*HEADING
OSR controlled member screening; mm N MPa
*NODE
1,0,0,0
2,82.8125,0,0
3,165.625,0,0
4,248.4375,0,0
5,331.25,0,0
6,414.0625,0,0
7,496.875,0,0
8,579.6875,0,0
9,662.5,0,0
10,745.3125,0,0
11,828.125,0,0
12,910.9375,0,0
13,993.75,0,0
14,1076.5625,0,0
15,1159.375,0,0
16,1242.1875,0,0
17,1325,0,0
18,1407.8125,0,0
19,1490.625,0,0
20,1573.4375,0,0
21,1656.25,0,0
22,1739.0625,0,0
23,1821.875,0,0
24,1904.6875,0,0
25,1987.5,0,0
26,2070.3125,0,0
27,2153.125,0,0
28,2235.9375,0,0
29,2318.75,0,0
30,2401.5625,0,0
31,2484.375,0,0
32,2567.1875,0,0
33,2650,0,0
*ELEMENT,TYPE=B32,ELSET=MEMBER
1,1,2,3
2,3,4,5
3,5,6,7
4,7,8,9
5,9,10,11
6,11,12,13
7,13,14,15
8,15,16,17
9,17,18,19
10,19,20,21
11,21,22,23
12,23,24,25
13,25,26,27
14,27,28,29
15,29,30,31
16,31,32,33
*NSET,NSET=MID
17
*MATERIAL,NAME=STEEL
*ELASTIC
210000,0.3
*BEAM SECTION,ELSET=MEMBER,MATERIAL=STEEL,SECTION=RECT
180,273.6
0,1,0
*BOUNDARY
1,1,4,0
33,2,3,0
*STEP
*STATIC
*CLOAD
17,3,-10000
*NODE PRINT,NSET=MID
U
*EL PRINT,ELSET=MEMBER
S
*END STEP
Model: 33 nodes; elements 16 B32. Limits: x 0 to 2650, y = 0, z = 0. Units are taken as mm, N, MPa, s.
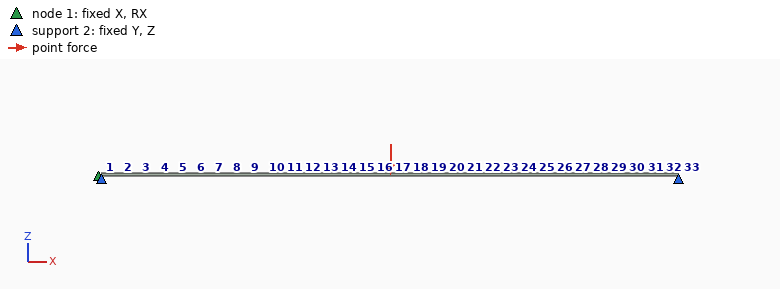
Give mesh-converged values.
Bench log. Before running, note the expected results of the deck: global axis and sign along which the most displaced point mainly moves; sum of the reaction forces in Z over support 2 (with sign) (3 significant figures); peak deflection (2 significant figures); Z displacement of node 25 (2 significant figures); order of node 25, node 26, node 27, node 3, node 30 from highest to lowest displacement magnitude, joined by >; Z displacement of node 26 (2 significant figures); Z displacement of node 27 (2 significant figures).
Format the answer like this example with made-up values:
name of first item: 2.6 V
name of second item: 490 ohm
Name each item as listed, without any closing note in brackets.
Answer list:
global axis and sign along which the most displaced point mainly moves: -Z
sum of the reaction forces in Z over support 2 (with sign): 10000 N
peak deflection: 0.062 mm
Z displacement of node 25: -0.042 mm
order of node 25, node 26, node 27, node 3, node 30 from highest to lowest displacement magnitude, joined by >: node 25 > node 26 > node 27 > node 30 > node 3
Z displacement of node 26: -0.038 mm
Z displacement of node 27: -0.033 mm
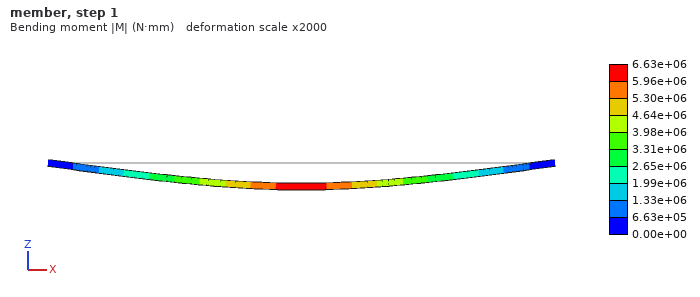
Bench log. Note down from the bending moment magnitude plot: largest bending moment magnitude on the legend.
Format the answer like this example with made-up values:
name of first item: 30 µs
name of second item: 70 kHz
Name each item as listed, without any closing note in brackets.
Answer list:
largest bending moment magnitude on the legend: 6.63e+06 N·mm
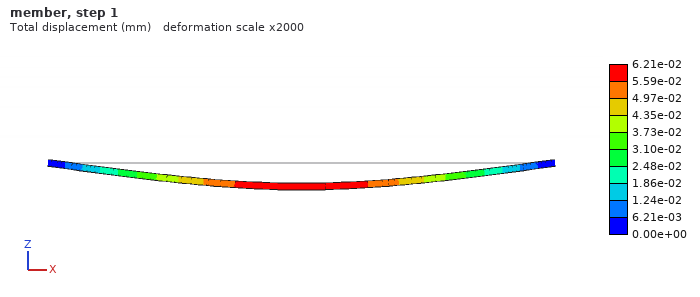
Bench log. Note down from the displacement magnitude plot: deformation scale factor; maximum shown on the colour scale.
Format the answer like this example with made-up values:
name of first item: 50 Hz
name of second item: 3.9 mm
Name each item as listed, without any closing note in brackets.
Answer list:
deformation scale factor: 2000
maximum shown on the colour scale: 6.21e-02 mm
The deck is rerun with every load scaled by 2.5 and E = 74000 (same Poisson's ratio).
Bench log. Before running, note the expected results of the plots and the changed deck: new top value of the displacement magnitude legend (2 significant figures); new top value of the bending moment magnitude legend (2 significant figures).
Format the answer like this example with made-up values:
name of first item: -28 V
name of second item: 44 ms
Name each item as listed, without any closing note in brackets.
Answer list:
new top value of the displacement magnitude legend: 0.44 mm
new top value of the bending moment magnitude legend: 1.7e+07 N·mm
